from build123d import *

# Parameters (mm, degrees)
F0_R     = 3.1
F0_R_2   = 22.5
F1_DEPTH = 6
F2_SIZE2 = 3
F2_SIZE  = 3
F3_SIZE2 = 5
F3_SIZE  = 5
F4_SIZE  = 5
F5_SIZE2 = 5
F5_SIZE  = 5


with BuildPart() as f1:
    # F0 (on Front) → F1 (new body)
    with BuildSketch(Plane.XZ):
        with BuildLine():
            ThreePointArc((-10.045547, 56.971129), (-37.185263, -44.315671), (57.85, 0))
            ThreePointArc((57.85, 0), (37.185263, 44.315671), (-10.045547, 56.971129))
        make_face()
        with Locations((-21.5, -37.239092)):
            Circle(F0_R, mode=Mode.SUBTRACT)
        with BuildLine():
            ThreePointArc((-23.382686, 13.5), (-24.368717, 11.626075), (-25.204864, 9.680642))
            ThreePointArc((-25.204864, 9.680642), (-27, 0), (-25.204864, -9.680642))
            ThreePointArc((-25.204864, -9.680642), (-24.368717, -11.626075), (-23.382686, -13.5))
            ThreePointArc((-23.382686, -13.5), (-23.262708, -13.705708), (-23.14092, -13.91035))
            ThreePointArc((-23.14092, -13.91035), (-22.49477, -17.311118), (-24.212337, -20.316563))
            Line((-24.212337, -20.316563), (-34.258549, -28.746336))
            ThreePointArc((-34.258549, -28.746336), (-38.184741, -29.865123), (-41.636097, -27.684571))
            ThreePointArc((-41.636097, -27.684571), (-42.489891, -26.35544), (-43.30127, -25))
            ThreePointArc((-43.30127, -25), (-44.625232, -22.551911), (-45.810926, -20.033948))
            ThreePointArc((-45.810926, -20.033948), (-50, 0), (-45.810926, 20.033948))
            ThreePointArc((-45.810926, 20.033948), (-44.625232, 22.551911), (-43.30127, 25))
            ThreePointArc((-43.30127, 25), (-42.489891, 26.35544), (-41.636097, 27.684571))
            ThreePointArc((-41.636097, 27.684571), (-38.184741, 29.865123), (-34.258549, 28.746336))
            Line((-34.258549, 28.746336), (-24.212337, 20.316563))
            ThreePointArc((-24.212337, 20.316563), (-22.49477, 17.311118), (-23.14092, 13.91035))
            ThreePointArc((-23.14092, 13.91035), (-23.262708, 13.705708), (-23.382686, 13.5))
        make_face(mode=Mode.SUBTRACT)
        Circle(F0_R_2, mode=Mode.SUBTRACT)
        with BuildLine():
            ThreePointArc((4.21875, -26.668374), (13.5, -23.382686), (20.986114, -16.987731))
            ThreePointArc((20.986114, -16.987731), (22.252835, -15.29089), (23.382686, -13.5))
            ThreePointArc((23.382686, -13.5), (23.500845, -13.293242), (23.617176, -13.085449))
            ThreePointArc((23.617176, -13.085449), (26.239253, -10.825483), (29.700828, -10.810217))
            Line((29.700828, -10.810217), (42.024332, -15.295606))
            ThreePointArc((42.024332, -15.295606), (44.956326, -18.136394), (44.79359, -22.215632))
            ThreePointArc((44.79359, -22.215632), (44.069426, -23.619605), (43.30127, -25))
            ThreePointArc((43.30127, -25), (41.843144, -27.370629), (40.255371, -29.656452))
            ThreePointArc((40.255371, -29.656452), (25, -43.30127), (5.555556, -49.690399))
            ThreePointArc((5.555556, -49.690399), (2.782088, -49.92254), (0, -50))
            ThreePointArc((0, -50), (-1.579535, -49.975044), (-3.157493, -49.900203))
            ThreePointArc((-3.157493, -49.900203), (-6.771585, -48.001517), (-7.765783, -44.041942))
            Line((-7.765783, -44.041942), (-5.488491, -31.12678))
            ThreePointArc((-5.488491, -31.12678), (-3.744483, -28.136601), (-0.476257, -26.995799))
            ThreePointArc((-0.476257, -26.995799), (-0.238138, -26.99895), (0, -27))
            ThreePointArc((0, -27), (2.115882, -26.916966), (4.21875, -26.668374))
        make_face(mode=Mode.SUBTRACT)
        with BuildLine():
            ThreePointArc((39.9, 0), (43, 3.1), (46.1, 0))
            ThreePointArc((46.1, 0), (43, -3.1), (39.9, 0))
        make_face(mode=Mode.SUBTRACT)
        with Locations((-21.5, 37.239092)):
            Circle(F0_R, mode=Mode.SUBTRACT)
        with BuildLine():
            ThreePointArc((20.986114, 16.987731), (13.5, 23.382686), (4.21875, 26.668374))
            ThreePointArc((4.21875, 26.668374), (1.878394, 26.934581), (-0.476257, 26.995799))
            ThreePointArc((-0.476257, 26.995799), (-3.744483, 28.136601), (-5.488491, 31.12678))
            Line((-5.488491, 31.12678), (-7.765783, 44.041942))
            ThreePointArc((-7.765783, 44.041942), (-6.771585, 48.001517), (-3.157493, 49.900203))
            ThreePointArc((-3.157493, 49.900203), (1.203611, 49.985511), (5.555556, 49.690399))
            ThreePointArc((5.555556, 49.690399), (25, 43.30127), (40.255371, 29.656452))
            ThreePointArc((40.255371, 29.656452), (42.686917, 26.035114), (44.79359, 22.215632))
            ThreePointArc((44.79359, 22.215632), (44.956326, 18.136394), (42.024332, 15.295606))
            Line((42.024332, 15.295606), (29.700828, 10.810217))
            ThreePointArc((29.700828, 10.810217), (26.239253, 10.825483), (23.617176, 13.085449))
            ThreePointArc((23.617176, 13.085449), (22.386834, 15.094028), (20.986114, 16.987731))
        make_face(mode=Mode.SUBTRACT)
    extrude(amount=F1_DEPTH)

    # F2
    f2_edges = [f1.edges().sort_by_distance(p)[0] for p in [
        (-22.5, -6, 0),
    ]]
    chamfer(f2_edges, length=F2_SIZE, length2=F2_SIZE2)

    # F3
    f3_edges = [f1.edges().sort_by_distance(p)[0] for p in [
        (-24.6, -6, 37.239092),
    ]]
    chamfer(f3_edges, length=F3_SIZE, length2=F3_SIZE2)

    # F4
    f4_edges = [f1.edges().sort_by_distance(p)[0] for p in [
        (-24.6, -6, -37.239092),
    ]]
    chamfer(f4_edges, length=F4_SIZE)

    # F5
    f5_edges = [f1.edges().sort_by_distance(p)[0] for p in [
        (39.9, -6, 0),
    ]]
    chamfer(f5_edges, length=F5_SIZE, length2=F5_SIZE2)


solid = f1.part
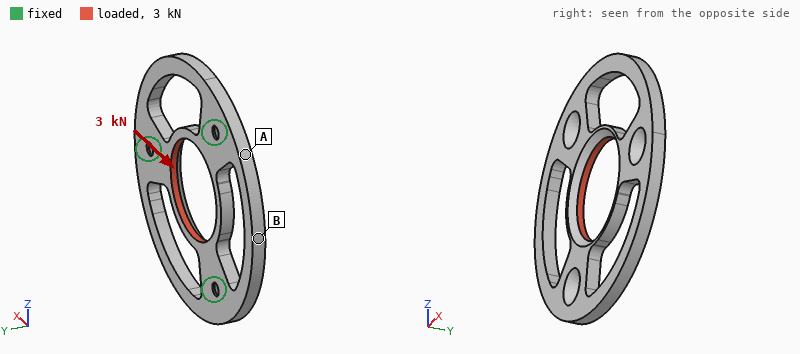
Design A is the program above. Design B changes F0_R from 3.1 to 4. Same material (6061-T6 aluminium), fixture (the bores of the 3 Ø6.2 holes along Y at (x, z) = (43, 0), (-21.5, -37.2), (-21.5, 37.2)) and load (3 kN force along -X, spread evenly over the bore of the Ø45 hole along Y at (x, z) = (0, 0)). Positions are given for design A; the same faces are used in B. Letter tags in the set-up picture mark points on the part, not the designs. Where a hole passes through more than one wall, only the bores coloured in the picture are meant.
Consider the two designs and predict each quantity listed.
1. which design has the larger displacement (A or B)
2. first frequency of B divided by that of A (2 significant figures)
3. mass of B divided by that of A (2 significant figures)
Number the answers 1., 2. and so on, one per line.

1. A
2. 1.0
3. 0.99
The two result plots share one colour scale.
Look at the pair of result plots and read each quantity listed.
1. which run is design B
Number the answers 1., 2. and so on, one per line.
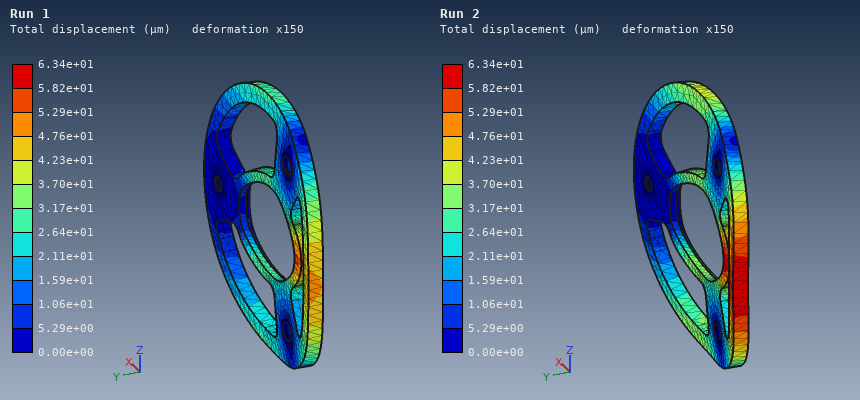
1. Run 1
